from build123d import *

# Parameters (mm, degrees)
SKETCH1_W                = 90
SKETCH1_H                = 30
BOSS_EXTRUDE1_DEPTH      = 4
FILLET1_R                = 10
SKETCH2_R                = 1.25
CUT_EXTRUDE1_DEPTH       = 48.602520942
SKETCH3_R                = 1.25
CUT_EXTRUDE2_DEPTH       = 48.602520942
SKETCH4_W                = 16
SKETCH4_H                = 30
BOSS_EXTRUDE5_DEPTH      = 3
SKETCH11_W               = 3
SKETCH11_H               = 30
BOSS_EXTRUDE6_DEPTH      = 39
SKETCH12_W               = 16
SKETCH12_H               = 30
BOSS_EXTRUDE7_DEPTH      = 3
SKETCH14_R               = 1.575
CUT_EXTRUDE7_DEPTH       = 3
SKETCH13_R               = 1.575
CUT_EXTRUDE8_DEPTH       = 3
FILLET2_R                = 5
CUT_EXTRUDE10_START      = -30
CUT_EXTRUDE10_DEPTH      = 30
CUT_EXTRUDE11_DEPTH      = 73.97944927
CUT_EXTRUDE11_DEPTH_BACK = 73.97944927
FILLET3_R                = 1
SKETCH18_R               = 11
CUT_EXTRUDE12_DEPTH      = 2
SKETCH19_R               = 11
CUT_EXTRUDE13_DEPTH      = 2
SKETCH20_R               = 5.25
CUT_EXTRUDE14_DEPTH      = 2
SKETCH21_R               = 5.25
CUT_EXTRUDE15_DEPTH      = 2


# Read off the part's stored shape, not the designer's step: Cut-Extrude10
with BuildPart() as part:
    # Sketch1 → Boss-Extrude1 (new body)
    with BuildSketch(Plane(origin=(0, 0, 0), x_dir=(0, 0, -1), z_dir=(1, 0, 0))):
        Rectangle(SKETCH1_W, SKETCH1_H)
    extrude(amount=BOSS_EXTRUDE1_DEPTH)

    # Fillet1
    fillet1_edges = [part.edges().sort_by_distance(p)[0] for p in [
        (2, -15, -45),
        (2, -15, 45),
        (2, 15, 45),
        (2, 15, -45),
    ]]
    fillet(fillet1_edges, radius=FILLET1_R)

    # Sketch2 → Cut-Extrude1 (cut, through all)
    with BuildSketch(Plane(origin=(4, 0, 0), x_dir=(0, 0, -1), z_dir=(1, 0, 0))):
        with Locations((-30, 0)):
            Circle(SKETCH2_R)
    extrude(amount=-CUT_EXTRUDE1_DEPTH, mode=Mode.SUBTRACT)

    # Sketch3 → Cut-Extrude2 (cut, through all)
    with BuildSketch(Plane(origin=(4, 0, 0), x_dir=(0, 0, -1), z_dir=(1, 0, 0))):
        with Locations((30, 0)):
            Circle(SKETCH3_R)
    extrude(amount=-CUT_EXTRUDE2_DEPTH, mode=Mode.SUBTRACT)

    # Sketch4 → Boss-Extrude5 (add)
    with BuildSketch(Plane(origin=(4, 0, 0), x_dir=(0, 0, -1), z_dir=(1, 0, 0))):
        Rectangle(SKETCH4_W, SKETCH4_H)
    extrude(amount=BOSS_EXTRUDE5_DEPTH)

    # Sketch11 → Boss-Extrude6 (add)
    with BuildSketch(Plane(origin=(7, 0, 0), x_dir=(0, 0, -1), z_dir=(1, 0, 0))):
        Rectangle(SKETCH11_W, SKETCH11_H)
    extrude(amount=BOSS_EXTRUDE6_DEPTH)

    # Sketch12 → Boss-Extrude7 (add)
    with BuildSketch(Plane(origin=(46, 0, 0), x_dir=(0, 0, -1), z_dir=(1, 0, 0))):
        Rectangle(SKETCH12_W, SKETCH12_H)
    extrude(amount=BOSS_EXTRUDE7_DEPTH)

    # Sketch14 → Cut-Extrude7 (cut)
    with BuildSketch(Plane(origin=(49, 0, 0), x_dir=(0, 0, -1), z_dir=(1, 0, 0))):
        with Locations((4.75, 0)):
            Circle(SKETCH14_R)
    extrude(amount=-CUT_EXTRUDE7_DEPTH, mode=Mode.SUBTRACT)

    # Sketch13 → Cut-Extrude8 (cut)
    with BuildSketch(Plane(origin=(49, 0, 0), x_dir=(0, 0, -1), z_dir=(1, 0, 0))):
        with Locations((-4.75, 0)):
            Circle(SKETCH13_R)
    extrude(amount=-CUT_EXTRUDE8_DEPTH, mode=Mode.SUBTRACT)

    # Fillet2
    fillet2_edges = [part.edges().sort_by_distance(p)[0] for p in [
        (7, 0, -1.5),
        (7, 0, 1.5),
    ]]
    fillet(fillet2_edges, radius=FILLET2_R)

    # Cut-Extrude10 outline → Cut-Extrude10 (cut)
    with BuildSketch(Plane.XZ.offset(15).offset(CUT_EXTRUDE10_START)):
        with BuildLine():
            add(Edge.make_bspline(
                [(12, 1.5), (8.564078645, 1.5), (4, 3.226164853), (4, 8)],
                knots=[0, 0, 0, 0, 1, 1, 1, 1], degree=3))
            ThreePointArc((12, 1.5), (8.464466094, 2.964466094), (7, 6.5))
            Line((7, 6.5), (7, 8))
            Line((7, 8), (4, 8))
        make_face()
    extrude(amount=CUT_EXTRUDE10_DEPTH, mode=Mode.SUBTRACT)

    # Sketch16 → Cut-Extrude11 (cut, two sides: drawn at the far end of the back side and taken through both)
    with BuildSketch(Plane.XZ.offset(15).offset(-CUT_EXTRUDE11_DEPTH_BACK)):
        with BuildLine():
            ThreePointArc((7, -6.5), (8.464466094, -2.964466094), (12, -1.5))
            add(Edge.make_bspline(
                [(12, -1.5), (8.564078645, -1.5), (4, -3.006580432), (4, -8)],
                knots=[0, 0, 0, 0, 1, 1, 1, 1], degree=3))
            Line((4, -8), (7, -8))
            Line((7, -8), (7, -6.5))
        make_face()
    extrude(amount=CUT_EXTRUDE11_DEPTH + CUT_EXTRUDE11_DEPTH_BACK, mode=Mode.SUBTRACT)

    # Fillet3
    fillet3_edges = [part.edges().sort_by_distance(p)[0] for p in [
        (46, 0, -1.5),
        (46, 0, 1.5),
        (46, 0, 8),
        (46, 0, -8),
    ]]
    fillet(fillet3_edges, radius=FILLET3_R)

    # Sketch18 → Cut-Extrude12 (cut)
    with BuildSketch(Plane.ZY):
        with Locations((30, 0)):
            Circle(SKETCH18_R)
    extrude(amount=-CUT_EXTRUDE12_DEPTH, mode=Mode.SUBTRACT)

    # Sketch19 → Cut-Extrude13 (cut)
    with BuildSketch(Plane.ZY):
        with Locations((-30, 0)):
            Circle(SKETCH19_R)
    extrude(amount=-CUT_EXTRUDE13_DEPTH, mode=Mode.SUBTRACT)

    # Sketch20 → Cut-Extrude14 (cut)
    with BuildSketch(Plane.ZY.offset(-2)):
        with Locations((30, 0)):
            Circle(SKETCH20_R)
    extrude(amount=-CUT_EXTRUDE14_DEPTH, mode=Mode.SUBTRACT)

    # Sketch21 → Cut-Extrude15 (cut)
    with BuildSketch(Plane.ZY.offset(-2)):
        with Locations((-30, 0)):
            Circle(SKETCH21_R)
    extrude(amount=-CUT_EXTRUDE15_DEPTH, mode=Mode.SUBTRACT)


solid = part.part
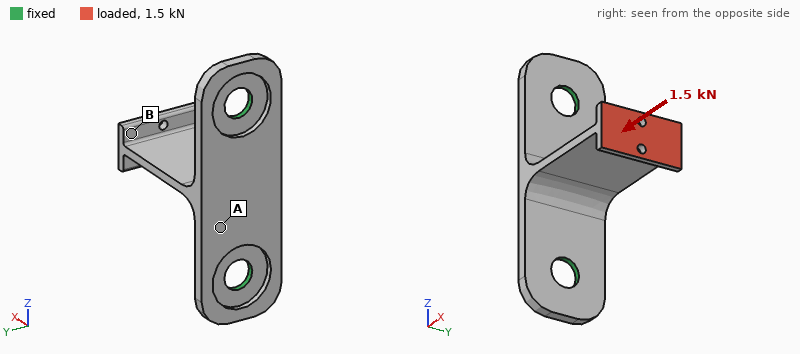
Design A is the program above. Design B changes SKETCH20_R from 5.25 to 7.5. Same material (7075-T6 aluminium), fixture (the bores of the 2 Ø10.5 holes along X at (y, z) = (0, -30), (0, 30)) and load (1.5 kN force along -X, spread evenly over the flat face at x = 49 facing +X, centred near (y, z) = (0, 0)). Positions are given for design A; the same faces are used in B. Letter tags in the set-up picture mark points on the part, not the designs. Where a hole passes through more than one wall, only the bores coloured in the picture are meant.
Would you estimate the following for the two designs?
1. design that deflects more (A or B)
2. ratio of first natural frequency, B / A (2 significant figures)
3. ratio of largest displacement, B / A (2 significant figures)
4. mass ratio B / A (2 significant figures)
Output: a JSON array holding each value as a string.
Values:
["A", "1.0", "0.92", "0.99"]
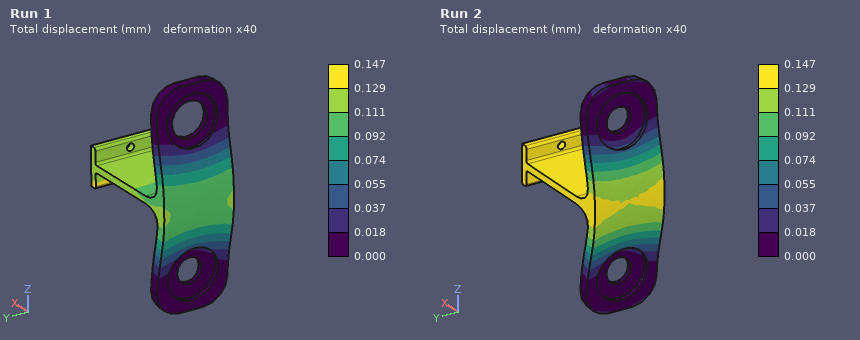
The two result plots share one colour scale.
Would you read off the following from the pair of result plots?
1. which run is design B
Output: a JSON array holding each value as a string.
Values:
["Run 1"]
